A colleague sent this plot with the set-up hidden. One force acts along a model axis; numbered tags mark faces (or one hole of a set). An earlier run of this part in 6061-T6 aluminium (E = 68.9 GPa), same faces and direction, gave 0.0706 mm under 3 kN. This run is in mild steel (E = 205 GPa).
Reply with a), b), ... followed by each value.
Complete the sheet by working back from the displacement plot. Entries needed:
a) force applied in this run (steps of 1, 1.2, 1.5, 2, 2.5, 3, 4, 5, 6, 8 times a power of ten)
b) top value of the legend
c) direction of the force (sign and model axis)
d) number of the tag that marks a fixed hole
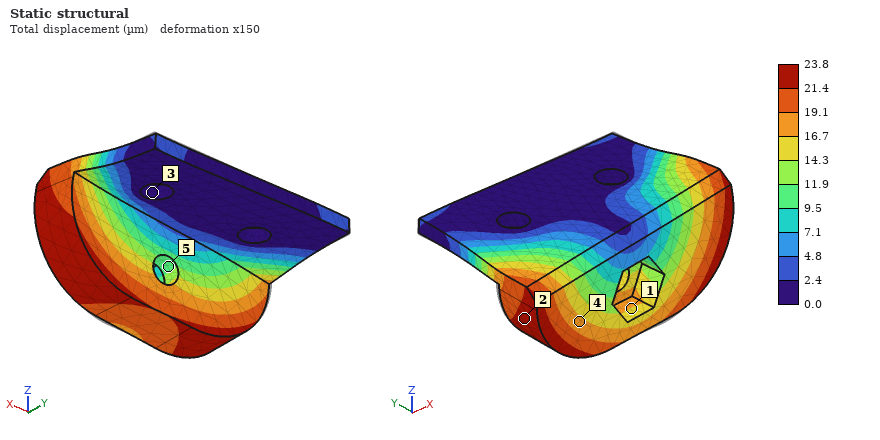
a) 3 kN
b) 23.8 µm
c) +X
d) 3
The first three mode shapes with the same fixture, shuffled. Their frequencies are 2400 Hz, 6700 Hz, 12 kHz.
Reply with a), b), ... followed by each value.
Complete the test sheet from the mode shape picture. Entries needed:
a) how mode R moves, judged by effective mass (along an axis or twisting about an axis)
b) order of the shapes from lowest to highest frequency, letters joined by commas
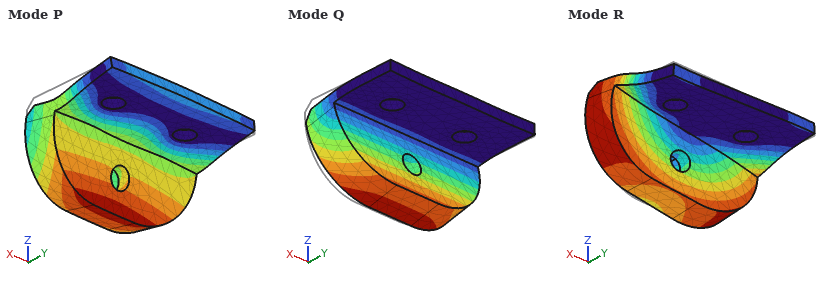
a) along X
b) Q, R, P
